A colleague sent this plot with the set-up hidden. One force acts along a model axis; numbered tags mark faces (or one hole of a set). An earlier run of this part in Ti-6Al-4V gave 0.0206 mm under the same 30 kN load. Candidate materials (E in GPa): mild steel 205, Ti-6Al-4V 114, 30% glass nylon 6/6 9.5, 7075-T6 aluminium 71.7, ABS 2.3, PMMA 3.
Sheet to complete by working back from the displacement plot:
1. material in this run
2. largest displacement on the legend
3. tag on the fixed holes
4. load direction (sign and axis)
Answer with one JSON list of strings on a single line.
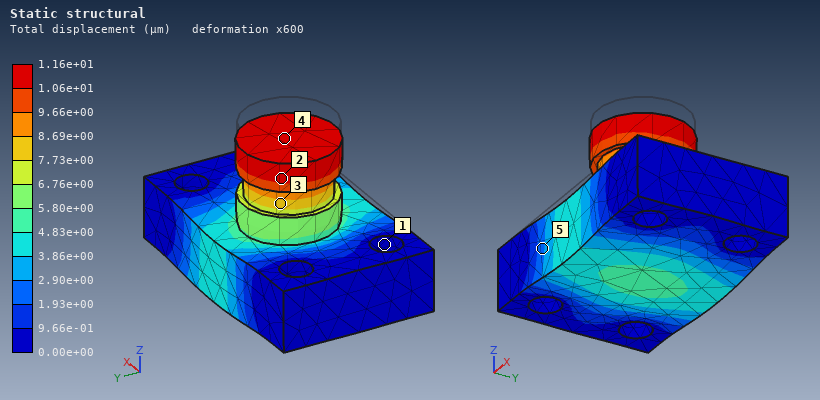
["mild steel", "1.16e+01 µm", "1", "-Z"]
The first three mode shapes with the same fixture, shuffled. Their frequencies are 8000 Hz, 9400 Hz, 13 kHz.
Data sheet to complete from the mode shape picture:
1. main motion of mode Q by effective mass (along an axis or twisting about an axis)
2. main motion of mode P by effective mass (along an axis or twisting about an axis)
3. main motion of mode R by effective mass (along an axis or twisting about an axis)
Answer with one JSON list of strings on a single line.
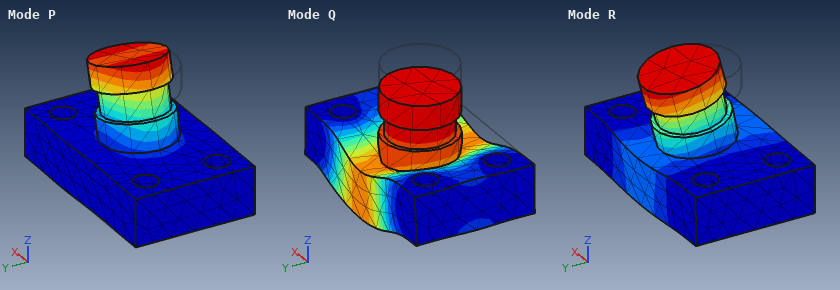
["along Z", "along X", "along Y"]
